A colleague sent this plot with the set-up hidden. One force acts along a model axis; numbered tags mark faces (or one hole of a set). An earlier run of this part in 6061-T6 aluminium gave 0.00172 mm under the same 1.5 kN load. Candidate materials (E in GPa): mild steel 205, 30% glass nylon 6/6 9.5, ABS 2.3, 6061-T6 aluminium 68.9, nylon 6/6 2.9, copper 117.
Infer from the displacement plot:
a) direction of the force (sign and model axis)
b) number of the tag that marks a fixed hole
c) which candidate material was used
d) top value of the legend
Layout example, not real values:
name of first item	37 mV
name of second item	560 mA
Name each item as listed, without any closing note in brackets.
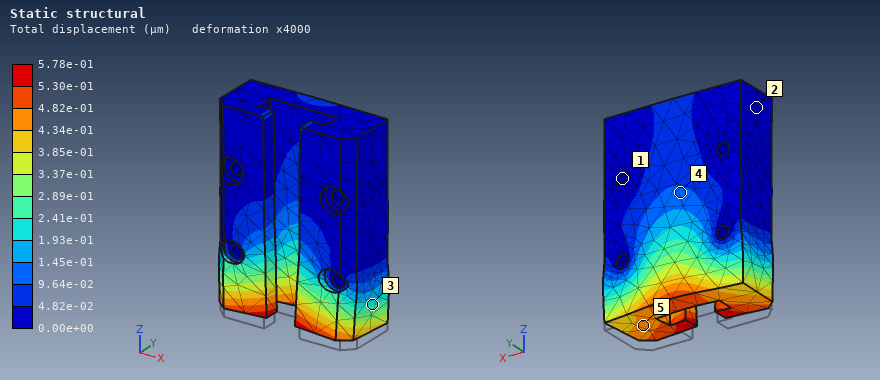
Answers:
direction of the force	+Z
number of the tag that marks a fixed hole	1
which candidate material was used	mild steel
top value of the legend	5.78e-01 µm
